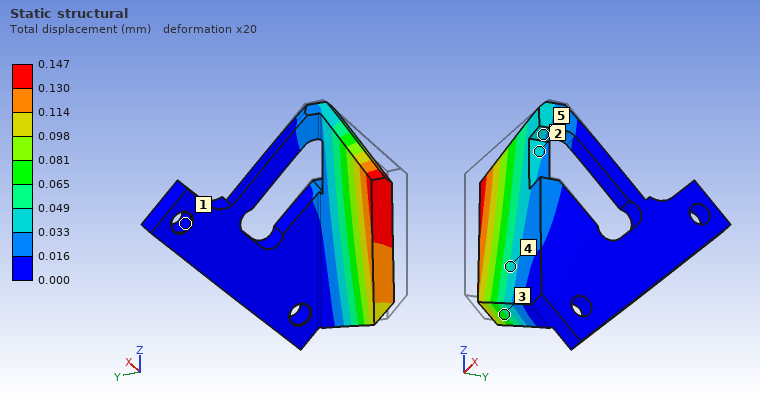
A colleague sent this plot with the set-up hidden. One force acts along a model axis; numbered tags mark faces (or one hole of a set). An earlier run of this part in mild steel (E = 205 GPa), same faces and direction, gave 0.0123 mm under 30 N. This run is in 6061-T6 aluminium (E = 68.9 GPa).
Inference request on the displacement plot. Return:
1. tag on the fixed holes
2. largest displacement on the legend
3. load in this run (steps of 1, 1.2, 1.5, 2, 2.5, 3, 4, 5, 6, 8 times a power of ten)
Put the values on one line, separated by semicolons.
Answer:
1; 0.147 mm; 120 N
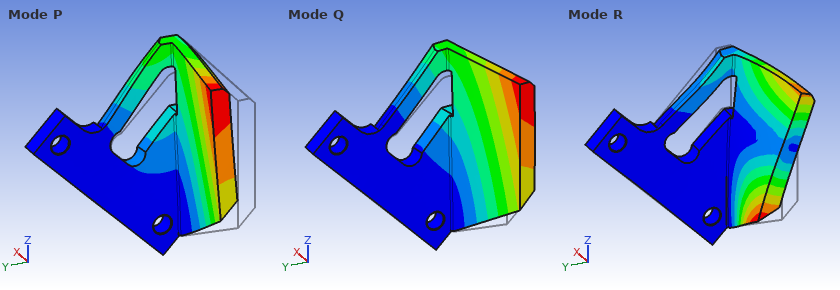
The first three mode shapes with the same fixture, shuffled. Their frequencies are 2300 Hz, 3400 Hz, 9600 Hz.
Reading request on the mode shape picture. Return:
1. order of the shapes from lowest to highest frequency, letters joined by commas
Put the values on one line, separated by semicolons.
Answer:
Q, P, R
